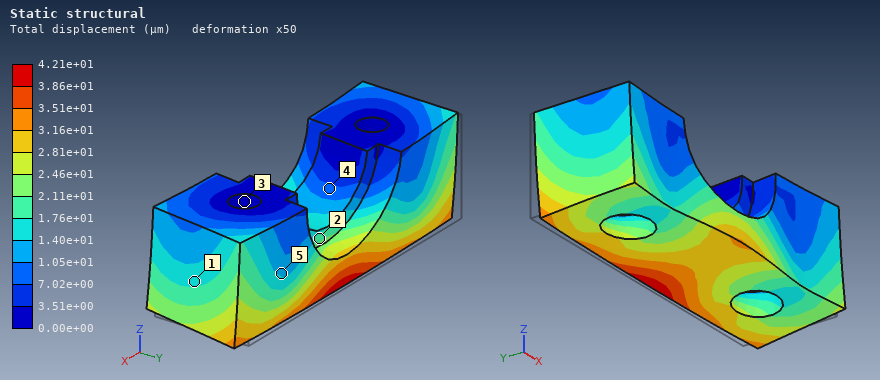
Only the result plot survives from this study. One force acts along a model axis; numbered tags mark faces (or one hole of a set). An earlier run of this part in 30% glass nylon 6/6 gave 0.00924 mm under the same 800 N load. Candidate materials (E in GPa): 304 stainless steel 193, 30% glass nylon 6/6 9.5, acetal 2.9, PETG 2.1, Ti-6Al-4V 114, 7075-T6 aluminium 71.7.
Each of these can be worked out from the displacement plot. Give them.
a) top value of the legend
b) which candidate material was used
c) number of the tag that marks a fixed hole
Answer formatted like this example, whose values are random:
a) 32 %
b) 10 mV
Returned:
a) 4.21e+01 µm
b) PETG
c) 3
